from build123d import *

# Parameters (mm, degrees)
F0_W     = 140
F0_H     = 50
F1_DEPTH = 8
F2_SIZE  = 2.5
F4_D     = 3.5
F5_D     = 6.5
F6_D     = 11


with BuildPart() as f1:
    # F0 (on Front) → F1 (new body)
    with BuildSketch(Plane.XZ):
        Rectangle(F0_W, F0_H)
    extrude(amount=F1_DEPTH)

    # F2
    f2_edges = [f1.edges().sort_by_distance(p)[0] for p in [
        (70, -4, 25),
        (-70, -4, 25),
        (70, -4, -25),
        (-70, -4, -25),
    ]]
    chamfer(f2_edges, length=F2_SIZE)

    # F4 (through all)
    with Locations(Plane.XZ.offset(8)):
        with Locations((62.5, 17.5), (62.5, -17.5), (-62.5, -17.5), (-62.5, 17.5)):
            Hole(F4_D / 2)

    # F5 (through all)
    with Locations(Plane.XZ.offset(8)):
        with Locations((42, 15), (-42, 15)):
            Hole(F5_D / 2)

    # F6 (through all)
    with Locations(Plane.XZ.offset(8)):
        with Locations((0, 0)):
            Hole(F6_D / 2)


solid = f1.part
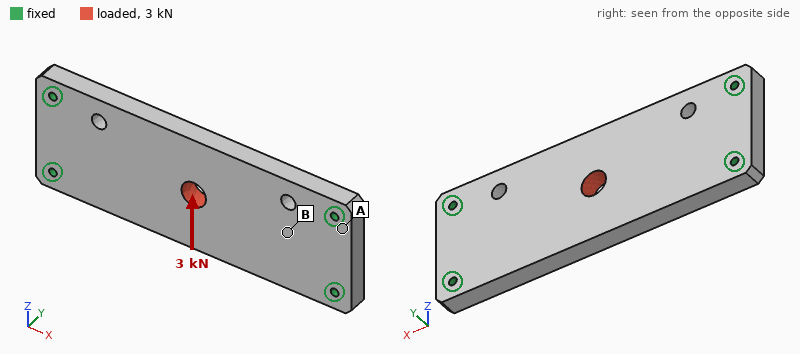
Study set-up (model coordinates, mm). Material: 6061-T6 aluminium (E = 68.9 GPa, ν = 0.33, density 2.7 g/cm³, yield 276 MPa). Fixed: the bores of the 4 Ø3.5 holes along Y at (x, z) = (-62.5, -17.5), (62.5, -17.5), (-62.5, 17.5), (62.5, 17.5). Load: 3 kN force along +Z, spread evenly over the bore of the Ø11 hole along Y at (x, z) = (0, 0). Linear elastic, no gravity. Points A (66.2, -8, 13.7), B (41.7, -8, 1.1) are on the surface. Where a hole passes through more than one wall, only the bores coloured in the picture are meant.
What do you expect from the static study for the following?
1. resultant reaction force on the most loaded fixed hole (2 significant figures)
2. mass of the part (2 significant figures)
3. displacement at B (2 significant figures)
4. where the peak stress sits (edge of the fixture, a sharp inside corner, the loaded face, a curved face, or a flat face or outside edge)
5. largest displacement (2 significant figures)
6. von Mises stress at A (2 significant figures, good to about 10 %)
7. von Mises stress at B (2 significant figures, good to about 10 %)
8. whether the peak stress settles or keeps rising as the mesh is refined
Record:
1.4 kN
150 g
5.8 µm
edge of the fixture
18 µm
4.8 MPa
11 MPa
keeps rising
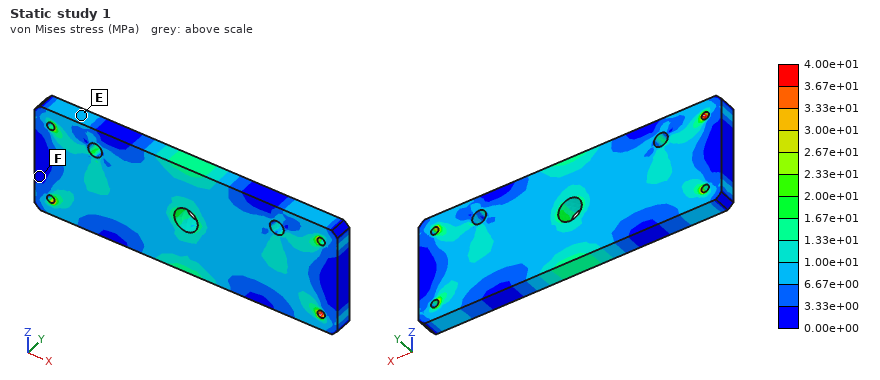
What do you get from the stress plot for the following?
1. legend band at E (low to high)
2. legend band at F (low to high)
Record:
6.67e+00 to 1.00e+01 MPa
0.00e+00 to 3.33e+00 MPa
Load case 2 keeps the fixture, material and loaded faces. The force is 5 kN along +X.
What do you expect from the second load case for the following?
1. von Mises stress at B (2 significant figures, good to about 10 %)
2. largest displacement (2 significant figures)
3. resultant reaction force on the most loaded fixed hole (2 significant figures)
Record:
5.5 MPa
8.8 µm
1.3 kN
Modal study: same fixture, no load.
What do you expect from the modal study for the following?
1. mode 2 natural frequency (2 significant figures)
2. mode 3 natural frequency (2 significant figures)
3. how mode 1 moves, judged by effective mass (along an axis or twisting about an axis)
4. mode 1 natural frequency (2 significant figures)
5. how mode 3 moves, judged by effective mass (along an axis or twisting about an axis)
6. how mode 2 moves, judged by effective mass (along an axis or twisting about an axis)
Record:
4500 Hz
6400 Hz
along Y
2400 Hz
twisting about Z
twisting about X
